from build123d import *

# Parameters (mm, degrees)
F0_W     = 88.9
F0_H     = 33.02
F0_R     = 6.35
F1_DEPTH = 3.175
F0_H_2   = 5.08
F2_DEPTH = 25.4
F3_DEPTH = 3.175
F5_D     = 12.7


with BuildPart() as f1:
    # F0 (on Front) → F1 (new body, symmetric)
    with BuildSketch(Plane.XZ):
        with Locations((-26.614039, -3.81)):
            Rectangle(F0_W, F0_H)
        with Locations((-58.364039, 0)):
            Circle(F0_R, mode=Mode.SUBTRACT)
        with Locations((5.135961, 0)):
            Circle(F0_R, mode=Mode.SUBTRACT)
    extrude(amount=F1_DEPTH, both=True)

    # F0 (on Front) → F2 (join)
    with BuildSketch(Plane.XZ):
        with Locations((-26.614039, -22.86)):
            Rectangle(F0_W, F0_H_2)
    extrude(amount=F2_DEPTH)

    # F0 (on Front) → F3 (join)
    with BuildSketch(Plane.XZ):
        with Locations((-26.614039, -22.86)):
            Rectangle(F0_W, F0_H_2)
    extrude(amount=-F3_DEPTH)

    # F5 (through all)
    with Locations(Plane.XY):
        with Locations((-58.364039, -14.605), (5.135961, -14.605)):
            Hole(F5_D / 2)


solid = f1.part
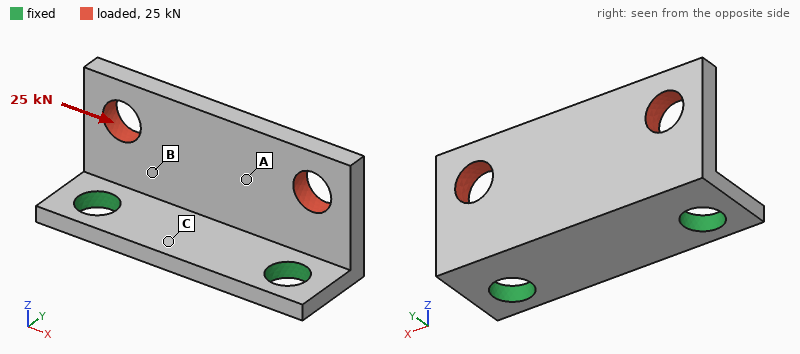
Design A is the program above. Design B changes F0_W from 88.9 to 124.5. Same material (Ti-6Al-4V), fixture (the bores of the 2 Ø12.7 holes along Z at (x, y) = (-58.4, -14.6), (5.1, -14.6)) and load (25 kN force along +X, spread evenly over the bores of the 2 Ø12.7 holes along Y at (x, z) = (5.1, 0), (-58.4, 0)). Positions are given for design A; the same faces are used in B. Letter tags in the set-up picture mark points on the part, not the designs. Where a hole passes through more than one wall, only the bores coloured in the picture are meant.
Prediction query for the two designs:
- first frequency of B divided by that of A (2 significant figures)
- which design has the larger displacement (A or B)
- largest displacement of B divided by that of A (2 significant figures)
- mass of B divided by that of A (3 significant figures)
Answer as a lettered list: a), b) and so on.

a) 0.94
b) B
c) 1.1
d) 1.44
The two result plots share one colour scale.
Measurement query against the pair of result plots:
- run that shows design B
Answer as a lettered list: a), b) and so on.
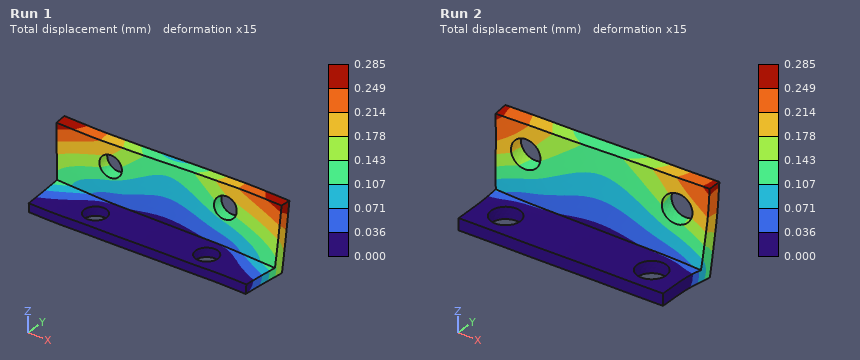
a) Run 1
